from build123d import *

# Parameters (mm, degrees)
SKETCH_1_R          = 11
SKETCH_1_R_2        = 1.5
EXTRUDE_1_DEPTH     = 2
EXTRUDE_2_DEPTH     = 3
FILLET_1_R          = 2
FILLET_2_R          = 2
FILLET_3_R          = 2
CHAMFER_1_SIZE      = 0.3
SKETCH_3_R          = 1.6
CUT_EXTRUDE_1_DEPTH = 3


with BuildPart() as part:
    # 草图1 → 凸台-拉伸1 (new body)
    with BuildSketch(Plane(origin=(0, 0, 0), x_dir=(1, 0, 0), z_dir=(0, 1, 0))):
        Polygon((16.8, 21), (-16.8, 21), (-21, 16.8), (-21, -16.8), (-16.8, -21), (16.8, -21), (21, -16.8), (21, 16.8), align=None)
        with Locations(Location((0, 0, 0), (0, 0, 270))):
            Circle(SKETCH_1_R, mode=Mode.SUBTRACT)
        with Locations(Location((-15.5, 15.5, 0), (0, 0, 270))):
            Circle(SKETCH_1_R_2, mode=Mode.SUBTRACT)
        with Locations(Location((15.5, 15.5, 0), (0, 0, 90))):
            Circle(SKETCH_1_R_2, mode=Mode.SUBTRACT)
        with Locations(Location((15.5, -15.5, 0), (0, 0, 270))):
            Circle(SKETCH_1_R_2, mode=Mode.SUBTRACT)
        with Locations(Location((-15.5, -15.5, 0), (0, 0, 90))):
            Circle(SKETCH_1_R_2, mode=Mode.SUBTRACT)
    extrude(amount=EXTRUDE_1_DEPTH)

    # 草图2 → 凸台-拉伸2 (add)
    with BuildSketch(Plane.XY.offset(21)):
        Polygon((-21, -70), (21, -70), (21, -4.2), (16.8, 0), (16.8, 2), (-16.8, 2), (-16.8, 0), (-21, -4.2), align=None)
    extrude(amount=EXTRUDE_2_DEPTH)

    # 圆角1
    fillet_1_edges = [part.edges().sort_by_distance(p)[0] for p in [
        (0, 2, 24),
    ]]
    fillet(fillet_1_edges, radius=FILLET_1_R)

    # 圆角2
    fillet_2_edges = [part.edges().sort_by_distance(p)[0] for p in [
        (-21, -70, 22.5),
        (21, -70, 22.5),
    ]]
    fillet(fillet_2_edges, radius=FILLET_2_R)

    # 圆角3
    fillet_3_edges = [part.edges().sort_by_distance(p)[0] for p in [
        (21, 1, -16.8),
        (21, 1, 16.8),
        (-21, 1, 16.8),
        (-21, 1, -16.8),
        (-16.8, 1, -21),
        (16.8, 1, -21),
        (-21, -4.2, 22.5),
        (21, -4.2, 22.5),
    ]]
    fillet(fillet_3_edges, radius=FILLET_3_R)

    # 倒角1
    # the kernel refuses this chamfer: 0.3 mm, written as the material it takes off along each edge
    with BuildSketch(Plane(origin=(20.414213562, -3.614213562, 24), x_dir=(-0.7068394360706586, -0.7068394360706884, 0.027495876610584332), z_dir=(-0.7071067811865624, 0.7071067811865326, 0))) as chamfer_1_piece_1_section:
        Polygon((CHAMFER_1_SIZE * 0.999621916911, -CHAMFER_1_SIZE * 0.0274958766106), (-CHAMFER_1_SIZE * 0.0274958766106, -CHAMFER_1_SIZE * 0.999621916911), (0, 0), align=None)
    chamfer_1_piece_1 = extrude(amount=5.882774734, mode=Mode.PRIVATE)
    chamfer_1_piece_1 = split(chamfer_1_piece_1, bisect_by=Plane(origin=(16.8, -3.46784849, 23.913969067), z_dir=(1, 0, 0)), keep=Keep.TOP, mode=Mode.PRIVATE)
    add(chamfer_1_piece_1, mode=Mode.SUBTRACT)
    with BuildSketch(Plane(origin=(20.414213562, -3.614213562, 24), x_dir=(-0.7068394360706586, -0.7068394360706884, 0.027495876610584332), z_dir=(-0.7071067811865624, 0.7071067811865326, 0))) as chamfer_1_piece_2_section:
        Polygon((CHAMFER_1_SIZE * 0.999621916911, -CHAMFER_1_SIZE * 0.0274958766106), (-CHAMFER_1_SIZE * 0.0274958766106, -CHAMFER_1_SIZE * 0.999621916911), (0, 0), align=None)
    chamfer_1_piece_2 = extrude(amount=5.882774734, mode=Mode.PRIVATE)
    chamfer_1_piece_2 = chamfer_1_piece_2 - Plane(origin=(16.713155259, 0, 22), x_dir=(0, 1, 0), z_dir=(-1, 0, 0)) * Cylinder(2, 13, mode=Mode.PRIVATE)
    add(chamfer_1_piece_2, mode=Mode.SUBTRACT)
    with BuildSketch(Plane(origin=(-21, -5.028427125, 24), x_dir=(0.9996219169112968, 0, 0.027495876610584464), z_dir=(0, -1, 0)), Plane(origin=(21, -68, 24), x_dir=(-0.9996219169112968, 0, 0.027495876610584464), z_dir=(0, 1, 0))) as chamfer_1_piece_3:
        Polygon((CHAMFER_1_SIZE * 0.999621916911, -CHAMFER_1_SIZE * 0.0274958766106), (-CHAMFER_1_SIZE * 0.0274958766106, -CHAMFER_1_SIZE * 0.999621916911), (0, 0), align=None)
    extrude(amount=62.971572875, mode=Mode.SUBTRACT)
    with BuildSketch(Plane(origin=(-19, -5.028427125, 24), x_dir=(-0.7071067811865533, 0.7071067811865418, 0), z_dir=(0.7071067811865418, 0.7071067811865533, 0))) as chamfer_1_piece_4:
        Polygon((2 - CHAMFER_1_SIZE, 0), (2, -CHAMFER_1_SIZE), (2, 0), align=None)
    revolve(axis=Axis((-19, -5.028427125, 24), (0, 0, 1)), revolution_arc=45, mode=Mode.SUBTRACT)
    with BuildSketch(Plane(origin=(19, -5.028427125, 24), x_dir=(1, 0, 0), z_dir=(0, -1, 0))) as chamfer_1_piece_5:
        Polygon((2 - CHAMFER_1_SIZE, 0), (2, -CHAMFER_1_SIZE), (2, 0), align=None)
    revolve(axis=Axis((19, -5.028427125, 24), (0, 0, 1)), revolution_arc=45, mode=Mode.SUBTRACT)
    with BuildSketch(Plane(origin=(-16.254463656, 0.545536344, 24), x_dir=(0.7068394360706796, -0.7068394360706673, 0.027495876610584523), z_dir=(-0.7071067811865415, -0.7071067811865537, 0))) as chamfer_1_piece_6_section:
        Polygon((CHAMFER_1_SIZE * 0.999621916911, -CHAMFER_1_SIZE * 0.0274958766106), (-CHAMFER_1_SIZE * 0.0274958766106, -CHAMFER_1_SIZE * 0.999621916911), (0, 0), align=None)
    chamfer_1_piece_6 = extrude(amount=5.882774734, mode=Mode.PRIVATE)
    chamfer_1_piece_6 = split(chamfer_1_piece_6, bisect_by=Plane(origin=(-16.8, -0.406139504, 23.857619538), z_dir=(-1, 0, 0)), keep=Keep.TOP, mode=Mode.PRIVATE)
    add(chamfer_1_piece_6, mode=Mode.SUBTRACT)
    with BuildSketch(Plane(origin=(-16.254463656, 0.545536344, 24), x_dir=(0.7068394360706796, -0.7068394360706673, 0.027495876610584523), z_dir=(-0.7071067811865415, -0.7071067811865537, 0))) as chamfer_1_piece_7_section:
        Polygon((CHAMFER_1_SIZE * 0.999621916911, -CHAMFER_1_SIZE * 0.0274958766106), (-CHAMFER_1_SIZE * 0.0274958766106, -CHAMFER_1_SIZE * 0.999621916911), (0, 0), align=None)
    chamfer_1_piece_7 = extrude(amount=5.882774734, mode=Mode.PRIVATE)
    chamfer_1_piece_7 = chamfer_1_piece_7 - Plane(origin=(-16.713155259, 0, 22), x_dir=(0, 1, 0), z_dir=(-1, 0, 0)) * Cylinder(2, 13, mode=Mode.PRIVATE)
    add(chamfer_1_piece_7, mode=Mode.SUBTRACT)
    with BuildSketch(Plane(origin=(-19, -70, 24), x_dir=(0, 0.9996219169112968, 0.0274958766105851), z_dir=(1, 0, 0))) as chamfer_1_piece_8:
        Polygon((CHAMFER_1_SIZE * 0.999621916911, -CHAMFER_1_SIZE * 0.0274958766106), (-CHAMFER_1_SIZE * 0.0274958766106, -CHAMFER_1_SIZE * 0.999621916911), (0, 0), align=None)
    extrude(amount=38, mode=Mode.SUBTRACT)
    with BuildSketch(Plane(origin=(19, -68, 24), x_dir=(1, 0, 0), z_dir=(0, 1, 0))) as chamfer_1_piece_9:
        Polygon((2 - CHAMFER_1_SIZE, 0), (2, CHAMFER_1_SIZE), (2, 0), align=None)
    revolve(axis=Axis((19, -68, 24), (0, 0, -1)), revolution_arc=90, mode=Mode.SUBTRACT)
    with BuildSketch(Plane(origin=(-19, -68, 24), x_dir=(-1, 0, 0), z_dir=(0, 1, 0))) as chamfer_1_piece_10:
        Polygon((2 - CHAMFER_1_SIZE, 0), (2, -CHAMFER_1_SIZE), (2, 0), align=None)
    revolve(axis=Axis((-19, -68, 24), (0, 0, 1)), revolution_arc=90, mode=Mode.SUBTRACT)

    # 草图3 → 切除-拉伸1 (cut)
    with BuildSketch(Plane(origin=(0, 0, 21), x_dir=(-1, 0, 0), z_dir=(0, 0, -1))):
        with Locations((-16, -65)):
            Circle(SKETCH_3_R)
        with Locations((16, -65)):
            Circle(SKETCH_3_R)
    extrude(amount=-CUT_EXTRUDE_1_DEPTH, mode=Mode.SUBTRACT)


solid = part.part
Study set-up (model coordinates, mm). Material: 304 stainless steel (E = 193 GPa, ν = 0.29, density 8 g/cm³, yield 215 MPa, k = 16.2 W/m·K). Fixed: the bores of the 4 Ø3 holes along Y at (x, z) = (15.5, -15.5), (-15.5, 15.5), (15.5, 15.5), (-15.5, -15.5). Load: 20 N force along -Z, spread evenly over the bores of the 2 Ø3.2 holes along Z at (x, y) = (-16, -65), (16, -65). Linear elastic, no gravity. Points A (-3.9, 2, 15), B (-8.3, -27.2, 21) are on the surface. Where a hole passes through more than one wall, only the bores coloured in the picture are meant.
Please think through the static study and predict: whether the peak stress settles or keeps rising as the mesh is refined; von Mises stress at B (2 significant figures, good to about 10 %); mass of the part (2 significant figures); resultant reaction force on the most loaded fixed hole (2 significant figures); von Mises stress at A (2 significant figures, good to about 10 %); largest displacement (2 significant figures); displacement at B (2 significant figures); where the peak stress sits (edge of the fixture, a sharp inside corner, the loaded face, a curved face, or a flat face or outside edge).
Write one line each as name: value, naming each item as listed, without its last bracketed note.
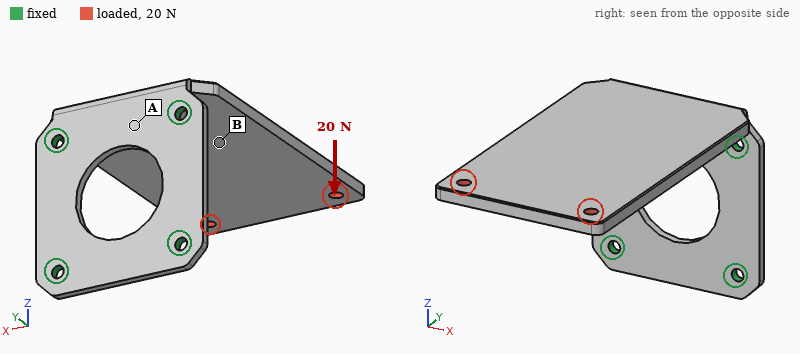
whether the peak stress settles or keeps rising as the mesh is refined: keeps rising
von Mises stress at B: 11 MPa
mass of the part: 92 g
resultant reaction force on the most loaded fixed hole: 11 N
von Mises stress at A: 23 MPa
largest displacement: 0.26 mm
displacement at B: 0.083 mm
where the peak stress sits: edge of the fixture
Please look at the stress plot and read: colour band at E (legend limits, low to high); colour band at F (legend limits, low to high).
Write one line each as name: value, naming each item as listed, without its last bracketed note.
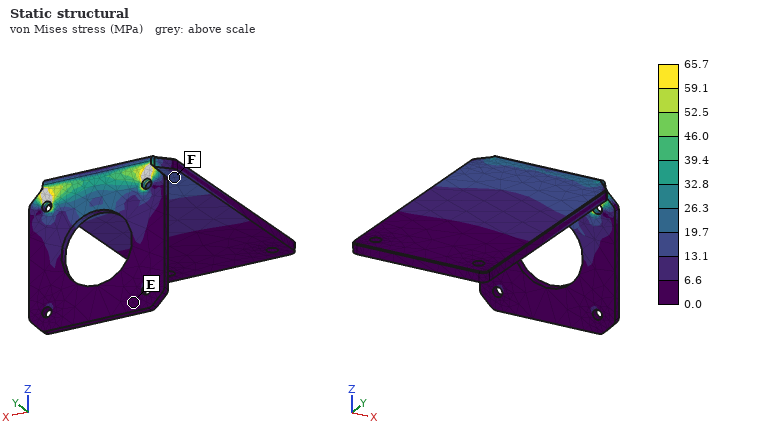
colour band at E: 0.0 to 6.6 MPa
colour band at F: 13.1 to 19.7 MPa
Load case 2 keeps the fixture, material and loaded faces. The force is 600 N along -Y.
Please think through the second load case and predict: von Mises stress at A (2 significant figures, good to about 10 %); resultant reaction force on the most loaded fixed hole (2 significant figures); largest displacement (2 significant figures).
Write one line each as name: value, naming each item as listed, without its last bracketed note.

von Mises stress at A: 32 MPa
resultant reaction force on the most loaded fixed hole: 310 N
largest displacement: 0.25 mm
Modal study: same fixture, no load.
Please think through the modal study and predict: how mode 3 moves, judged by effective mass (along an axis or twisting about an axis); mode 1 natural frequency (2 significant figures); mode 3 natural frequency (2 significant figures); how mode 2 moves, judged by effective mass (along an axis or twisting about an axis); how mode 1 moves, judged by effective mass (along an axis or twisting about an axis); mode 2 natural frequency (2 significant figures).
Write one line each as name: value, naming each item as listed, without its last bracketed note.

how mode 3 moves, judged by effective mass: along X
mode 1 natural frequency: 290 Hz
mode 3 natural frequency: 1800 Hz
how mode 2 moves, judged by effective mass: along X
how mode 1 moves, judged by effective mass: along Z
mode 2 natural frequency: 1400 Hz
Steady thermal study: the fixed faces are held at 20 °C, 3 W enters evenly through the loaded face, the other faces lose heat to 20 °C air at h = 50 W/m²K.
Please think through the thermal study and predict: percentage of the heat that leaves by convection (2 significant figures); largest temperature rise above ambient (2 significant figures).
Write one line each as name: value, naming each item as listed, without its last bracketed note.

percentage of the heat that leaves by convection: 97 %
largest temperature rise above ambient: 34 K
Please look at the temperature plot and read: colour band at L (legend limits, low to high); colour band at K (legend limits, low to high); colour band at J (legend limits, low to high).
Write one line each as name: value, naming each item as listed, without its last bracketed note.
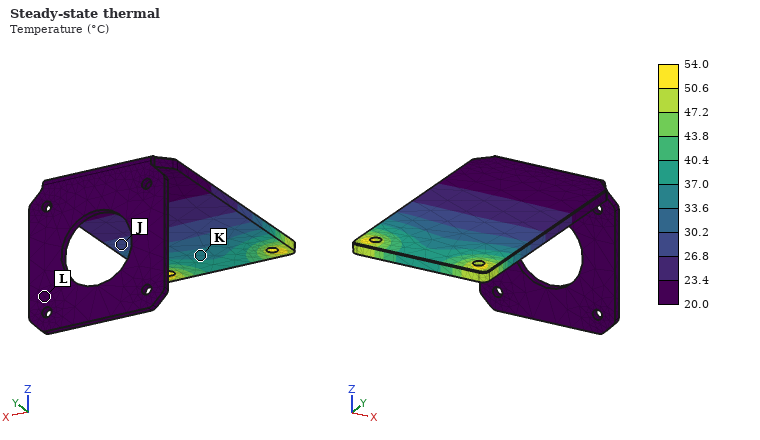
colour band at L: 20.0 to 23.4 °C
colour band at K: 33.6 to 37.0 °C
colour band at J: 26.8 to 30.2 °C
